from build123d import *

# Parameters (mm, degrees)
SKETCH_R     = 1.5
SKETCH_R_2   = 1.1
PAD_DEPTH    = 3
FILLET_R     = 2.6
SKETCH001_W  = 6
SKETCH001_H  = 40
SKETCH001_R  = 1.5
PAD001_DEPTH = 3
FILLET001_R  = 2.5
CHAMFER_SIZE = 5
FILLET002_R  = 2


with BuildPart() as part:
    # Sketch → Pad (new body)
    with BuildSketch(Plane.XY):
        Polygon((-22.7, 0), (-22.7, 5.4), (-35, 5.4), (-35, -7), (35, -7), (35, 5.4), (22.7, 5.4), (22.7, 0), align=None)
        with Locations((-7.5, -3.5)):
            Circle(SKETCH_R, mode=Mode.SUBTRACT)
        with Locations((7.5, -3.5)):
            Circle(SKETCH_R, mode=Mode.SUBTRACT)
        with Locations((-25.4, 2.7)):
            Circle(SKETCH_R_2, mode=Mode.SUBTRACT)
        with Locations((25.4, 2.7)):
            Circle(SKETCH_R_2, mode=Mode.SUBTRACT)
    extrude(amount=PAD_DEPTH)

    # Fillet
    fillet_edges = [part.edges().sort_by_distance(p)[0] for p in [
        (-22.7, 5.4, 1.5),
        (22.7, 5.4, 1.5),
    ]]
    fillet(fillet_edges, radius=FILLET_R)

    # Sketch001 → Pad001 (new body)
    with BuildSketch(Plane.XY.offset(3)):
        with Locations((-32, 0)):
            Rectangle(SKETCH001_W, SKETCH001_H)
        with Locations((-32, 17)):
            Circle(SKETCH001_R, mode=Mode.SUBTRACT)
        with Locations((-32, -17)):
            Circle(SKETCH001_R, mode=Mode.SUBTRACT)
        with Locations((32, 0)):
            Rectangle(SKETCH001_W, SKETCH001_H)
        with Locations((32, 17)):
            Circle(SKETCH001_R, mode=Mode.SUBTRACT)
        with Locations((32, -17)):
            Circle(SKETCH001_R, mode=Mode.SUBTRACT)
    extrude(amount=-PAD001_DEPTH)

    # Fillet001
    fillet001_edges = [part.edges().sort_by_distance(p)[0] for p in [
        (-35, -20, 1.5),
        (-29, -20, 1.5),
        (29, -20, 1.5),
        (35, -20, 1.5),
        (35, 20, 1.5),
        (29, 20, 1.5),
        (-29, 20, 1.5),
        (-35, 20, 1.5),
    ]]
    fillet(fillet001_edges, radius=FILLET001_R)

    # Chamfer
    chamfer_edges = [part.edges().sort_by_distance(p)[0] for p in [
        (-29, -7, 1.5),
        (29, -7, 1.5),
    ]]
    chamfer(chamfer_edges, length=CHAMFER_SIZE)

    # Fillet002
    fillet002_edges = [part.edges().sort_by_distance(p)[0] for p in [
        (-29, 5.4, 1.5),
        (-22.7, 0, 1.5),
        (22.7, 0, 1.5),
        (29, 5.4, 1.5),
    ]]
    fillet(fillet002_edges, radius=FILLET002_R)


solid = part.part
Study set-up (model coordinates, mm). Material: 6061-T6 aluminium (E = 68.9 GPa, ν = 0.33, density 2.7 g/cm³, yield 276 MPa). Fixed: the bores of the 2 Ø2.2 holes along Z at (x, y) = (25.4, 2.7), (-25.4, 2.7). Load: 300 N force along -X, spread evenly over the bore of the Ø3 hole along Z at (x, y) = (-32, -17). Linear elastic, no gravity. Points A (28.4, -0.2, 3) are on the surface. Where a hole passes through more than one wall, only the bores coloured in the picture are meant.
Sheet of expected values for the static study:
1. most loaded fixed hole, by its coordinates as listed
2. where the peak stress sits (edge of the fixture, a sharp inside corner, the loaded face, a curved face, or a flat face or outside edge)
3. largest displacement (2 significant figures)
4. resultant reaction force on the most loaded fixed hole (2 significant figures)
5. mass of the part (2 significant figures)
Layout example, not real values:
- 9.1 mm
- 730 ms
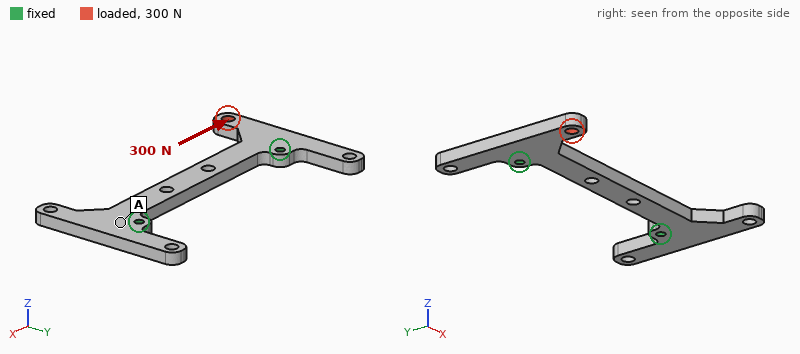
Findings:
- (25.4, 2.7)
- edge of the fixture
- 0.11 mm
- 290 N
- 7.4 g
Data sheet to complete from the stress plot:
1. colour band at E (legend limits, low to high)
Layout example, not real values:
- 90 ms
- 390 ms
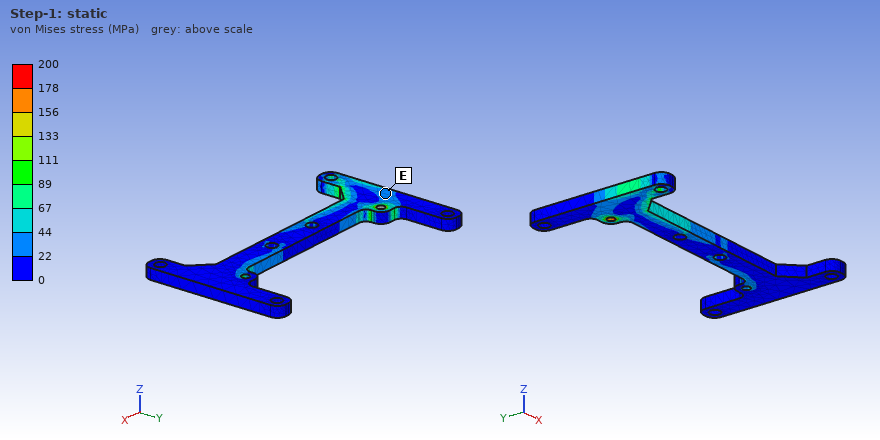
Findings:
- 22 to 44 MPa
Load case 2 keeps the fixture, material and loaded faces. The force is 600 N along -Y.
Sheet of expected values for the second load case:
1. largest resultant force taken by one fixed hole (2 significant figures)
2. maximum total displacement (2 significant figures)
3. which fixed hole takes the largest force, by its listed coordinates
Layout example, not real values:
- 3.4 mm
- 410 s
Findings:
- 660 N
- 58 µm
- (-25.4, 2.7)
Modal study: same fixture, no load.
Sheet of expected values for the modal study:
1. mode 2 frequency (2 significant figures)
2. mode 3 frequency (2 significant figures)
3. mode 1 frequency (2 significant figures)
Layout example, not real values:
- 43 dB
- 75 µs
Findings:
- 5600 Hz
- 5800 Hz
- 5000 Hz
